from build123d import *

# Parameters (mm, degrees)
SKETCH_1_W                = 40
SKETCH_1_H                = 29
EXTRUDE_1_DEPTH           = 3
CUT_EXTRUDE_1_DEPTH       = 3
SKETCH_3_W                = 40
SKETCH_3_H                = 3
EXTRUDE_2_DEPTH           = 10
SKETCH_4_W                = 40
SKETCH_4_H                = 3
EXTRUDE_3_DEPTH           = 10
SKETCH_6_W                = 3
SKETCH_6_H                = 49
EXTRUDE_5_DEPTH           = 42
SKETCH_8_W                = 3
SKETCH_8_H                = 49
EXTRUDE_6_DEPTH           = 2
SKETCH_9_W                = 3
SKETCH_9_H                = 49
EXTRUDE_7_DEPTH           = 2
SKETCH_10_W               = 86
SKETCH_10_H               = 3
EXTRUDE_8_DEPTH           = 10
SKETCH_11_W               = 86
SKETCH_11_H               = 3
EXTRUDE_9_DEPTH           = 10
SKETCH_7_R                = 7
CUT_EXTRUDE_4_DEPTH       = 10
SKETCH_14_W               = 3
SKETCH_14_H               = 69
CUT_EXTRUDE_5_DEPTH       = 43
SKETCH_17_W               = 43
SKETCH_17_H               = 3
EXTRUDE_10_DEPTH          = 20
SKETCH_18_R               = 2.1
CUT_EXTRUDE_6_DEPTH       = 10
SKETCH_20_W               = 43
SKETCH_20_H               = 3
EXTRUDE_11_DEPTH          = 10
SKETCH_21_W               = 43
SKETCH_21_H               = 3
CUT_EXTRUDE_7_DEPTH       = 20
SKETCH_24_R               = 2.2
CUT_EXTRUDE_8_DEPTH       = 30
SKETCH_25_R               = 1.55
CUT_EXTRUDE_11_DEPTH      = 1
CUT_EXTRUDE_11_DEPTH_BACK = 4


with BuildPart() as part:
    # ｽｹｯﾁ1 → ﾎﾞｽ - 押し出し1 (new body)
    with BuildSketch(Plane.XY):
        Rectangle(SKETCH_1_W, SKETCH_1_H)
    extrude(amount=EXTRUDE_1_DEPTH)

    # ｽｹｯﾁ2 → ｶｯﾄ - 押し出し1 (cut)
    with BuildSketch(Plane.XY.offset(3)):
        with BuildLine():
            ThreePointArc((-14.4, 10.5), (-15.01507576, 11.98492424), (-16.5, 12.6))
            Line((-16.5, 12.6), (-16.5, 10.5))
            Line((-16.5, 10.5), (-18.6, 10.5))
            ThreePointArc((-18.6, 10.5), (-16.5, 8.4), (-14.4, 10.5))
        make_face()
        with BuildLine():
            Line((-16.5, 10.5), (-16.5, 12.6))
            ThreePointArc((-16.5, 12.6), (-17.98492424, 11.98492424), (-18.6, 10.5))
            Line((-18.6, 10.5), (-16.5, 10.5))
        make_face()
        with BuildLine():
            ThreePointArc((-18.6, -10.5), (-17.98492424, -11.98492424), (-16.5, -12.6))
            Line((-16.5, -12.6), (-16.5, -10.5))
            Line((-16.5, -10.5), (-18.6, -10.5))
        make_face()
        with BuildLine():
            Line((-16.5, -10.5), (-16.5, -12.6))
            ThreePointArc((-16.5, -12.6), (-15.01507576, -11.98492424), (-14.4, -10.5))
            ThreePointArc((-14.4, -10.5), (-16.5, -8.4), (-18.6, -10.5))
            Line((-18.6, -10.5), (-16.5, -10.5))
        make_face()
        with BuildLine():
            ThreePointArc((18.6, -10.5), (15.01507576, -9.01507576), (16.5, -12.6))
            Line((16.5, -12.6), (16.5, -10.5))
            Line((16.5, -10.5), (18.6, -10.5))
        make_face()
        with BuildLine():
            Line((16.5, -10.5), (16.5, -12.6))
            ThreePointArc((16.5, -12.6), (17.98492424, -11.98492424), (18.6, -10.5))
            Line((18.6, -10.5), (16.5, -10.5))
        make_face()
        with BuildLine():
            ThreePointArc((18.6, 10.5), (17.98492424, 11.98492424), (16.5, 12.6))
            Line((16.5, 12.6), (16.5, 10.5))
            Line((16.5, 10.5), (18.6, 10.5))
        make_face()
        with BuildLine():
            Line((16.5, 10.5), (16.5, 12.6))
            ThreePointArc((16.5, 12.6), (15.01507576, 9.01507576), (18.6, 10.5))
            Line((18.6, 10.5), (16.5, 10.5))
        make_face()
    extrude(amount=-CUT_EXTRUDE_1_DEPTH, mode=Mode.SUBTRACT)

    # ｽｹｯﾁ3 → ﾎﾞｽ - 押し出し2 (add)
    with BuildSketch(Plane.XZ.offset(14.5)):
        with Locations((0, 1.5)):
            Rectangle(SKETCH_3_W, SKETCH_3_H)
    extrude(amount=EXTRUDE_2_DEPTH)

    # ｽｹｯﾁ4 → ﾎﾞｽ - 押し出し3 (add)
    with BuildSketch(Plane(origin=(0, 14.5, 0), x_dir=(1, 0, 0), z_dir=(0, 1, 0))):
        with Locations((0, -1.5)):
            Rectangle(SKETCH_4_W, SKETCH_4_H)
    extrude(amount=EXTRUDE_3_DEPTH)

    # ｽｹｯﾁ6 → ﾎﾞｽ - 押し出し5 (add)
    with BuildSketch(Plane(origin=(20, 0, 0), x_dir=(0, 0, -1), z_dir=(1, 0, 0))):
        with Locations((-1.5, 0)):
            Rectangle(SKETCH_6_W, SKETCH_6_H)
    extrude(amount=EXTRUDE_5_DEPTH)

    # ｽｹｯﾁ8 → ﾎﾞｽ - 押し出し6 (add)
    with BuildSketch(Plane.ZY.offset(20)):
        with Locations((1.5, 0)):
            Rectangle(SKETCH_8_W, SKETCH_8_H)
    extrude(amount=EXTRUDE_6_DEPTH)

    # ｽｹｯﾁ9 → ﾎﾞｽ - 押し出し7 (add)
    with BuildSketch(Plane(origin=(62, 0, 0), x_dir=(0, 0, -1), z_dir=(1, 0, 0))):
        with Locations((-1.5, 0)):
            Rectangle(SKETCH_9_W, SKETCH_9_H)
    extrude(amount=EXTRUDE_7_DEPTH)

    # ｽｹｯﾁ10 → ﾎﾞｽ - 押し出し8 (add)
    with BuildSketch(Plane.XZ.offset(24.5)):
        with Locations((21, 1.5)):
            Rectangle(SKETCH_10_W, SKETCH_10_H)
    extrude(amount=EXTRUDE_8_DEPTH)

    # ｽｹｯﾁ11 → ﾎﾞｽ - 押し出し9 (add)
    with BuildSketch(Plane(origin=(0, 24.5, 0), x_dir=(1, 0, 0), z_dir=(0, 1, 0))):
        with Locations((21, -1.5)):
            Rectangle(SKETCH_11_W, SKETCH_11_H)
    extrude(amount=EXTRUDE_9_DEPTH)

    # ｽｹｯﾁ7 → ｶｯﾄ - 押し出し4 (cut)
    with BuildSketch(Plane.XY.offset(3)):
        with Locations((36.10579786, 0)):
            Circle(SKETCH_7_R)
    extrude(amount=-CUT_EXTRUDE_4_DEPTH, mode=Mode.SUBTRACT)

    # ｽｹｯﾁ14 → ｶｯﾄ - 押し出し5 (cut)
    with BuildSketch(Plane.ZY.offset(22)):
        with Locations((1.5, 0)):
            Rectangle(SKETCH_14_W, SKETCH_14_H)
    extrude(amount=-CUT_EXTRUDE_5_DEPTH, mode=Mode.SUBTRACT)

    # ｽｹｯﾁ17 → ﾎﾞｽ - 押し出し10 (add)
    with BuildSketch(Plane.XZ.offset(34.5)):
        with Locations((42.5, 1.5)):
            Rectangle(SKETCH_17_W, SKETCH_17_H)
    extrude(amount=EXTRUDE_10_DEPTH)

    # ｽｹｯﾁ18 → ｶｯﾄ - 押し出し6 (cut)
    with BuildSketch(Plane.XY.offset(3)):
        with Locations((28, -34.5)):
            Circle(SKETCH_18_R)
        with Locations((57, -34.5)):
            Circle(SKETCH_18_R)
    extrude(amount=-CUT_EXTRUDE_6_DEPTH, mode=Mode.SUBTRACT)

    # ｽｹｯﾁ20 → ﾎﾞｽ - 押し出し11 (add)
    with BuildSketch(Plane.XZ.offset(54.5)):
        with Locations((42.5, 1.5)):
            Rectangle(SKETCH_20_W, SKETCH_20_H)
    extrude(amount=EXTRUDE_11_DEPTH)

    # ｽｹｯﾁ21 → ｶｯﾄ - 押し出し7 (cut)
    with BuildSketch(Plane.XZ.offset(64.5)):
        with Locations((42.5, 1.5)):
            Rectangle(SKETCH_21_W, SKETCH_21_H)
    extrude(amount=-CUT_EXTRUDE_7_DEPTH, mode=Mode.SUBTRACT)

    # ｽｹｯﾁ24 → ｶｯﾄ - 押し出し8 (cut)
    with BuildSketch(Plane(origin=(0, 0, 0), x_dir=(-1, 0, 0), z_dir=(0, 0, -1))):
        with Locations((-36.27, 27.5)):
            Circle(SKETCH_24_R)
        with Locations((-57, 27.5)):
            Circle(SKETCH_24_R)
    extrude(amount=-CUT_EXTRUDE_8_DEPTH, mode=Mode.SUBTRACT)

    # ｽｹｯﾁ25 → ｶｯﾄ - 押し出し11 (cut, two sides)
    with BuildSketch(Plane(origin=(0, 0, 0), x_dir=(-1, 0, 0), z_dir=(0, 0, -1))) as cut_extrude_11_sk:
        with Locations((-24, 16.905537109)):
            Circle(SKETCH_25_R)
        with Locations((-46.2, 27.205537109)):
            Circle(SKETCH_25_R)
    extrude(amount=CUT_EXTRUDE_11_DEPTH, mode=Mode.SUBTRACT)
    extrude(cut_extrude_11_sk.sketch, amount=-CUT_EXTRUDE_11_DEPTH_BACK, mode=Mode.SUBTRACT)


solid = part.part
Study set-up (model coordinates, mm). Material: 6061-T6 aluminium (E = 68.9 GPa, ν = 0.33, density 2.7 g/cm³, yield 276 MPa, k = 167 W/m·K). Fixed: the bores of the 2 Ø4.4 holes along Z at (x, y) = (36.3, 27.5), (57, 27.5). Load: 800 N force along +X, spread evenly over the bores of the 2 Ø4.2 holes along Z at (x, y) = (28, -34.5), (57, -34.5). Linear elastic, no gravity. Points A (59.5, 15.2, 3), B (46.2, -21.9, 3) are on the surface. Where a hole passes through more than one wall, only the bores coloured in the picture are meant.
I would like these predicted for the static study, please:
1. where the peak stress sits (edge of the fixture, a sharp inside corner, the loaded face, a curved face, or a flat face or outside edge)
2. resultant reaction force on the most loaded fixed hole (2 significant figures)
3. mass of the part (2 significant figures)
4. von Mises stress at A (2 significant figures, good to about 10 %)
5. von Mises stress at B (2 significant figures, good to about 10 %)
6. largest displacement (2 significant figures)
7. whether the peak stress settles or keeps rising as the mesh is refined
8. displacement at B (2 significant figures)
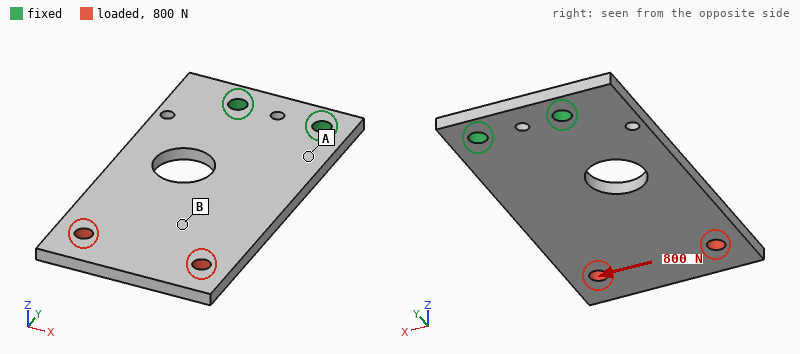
edge of the fixture
2.1 kN
26 g
44 MPa
14 MPa
0.13 mm
keeps rising
0.079 mm
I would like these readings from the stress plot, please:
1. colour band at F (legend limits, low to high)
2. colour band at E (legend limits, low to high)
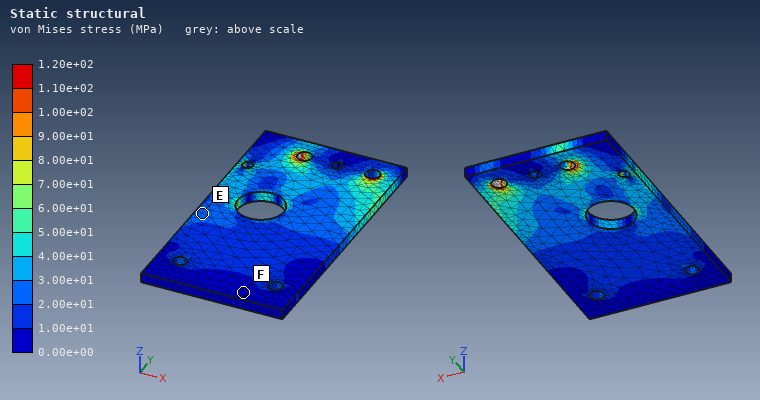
0.00e+00 to 1.00e+01 MPa
2.00e+01 to 3.00e+01 MPa
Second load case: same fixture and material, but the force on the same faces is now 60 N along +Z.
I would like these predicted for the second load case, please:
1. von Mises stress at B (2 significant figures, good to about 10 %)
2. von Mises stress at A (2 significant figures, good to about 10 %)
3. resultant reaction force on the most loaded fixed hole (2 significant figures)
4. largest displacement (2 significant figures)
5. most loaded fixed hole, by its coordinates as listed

11 MPa
51 MPa
43 N
0.99 mm
(36.3, 27.5)
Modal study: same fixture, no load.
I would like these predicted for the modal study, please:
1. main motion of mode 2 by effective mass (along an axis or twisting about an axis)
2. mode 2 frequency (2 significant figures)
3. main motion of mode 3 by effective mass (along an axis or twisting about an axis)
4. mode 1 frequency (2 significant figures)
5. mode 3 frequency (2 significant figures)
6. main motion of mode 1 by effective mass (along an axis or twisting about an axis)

twisting about Y
1600 Hz
along Z
460 Hz
2900 Hz
along Z
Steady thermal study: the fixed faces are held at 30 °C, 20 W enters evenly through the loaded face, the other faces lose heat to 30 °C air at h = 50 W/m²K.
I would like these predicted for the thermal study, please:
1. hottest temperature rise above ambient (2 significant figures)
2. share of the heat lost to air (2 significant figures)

49 K
42 %
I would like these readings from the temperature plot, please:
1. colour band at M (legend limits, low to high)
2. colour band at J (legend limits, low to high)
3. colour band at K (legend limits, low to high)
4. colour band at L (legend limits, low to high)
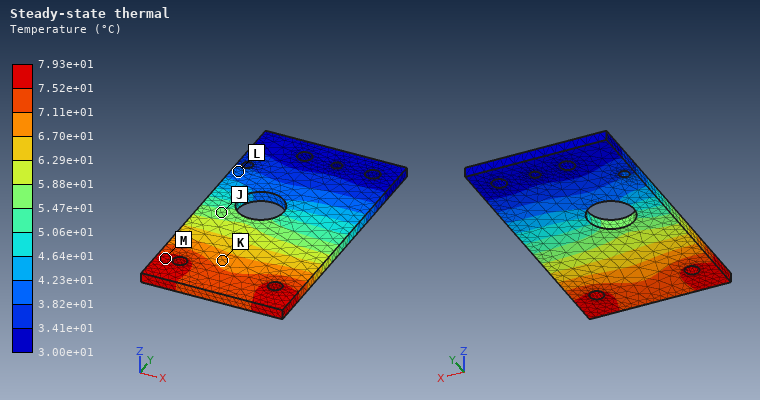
7.52e+01 to 7.93e+01 °C
5.47e+01 to 5.88e+01 °C
6.70e+01 to 7.11e+01 °C
3.82e+01 to 4.23e+01 °C
